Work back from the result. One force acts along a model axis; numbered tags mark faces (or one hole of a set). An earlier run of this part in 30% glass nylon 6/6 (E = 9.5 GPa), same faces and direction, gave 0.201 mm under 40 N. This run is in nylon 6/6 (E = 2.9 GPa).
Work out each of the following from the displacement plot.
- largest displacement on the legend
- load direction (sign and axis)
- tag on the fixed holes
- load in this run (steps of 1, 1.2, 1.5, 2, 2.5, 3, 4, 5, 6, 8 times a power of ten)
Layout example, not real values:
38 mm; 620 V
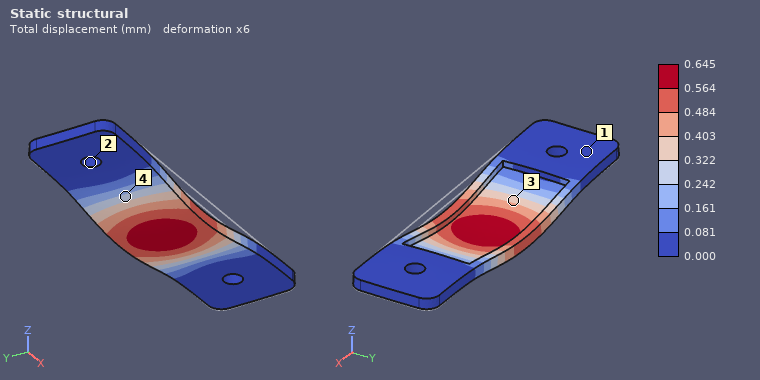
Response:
0.645 mm; -Z; 2; 40 N
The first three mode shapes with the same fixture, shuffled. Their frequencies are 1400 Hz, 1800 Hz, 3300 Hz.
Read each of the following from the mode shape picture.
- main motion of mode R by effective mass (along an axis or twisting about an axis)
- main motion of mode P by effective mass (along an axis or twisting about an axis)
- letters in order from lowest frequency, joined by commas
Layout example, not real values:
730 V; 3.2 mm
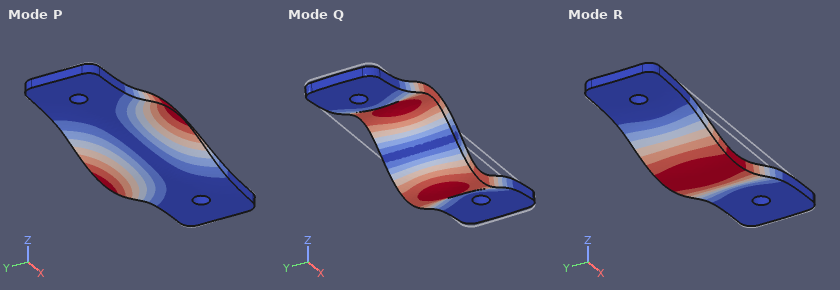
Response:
along Z; twisting about X; R, P, Q
